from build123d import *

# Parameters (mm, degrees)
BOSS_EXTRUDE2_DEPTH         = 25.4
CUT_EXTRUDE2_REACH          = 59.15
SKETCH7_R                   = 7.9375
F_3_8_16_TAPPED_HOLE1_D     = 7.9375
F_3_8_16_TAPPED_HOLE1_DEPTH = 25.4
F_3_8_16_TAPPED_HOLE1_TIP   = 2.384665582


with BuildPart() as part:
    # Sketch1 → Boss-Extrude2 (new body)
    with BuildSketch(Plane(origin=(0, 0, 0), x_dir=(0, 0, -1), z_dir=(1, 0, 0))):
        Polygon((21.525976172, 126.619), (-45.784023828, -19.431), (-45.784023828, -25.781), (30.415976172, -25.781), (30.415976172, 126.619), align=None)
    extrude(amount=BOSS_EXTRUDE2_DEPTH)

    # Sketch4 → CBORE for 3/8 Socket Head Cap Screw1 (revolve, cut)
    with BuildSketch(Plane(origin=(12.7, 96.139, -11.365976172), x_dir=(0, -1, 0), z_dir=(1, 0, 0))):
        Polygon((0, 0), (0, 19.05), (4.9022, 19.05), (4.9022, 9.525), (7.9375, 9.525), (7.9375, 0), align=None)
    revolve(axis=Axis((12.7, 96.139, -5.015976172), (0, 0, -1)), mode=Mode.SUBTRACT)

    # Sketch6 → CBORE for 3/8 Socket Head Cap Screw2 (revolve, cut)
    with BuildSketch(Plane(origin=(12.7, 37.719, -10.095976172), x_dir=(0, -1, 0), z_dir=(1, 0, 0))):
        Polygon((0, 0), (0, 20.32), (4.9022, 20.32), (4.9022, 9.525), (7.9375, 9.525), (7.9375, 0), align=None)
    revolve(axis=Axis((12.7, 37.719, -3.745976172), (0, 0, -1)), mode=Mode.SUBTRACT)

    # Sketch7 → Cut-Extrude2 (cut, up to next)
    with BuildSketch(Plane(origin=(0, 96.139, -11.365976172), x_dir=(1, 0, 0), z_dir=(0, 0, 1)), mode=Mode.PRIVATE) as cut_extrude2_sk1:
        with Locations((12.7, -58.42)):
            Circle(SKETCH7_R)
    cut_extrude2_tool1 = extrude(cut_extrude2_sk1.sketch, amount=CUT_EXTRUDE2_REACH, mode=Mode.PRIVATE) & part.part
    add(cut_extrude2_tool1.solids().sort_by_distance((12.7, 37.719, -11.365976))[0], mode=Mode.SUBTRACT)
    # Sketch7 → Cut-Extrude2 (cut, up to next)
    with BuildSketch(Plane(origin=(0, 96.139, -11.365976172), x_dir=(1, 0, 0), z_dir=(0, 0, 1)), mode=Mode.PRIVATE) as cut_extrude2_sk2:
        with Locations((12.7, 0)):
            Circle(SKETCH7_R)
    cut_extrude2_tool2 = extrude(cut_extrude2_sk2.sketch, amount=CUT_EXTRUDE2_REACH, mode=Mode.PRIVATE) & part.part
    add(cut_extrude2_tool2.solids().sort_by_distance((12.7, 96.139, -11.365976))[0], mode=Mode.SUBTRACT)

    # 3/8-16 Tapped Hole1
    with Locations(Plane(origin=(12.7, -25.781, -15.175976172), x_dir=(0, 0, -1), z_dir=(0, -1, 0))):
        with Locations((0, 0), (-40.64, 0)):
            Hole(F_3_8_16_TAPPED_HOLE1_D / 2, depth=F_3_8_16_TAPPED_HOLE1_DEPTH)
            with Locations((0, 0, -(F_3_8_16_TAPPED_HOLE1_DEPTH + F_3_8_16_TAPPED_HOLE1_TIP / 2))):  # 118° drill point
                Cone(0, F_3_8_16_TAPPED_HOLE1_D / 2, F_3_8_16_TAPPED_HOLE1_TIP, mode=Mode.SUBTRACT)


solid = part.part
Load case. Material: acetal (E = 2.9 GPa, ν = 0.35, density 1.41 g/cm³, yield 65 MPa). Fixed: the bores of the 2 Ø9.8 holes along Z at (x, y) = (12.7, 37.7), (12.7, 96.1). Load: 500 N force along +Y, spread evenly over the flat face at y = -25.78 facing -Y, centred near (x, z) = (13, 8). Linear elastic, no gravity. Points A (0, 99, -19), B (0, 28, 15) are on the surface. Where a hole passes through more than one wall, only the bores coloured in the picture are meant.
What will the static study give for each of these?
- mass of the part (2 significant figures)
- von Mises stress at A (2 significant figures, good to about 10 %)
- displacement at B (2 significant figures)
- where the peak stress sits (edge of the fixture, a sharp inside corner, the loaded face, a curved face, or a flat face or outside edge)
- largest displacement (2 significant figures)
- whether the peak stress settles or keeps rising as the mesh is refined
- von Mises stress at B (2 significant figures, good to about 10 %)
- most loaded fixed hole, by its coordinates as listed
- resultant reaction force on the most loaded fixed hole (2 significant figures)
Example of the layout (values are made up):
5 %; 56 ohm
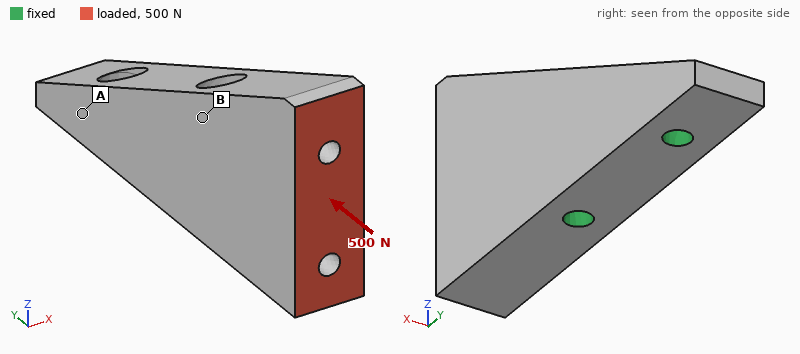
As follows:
220 g; 0.59 MPa; 0.045 mm; edge of the fixture; 0.13 mm; keeps rising; 1.7 MPa; (12.7, 96.1); 380 N
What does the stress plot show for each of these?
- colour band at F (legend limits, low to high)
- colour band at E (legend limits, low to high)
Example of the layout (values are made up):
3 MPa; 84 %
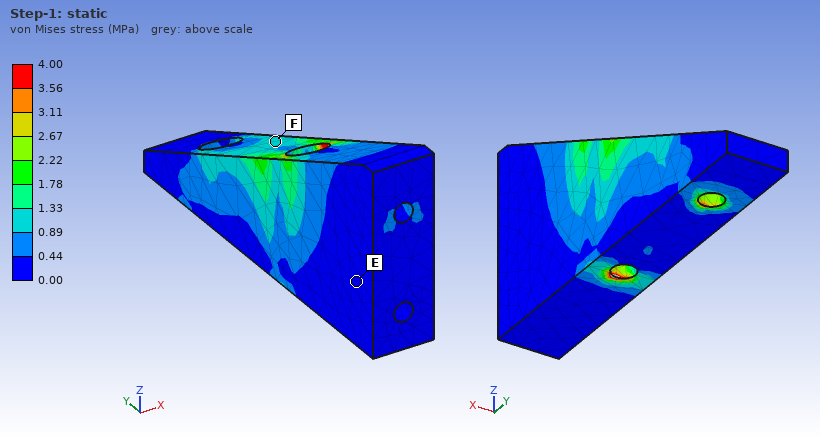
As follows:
0.89 to 1.33 MPa; 0.00 to 0.44 MPa
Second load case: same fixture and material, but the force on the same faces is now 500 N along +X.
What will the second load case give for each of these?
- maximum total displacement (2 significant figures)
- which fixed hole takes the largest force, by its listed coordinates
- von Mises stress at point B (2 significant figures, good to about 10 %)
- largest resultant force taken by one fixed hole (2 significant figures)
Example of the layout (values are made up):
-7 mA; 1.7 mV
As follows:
0.89 mm; (12.7, 37.7); 4.3 MPa; 850 N
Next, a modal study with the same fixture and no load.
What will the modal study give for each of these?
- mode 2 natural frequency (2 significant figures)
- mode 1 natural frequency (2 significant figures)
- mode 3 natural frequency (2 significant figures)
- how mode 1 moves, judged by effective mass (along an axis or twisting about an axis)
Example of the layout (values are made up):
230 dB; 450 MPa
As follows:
880 Hz; 540 Hz; 1200 Hz; along X
